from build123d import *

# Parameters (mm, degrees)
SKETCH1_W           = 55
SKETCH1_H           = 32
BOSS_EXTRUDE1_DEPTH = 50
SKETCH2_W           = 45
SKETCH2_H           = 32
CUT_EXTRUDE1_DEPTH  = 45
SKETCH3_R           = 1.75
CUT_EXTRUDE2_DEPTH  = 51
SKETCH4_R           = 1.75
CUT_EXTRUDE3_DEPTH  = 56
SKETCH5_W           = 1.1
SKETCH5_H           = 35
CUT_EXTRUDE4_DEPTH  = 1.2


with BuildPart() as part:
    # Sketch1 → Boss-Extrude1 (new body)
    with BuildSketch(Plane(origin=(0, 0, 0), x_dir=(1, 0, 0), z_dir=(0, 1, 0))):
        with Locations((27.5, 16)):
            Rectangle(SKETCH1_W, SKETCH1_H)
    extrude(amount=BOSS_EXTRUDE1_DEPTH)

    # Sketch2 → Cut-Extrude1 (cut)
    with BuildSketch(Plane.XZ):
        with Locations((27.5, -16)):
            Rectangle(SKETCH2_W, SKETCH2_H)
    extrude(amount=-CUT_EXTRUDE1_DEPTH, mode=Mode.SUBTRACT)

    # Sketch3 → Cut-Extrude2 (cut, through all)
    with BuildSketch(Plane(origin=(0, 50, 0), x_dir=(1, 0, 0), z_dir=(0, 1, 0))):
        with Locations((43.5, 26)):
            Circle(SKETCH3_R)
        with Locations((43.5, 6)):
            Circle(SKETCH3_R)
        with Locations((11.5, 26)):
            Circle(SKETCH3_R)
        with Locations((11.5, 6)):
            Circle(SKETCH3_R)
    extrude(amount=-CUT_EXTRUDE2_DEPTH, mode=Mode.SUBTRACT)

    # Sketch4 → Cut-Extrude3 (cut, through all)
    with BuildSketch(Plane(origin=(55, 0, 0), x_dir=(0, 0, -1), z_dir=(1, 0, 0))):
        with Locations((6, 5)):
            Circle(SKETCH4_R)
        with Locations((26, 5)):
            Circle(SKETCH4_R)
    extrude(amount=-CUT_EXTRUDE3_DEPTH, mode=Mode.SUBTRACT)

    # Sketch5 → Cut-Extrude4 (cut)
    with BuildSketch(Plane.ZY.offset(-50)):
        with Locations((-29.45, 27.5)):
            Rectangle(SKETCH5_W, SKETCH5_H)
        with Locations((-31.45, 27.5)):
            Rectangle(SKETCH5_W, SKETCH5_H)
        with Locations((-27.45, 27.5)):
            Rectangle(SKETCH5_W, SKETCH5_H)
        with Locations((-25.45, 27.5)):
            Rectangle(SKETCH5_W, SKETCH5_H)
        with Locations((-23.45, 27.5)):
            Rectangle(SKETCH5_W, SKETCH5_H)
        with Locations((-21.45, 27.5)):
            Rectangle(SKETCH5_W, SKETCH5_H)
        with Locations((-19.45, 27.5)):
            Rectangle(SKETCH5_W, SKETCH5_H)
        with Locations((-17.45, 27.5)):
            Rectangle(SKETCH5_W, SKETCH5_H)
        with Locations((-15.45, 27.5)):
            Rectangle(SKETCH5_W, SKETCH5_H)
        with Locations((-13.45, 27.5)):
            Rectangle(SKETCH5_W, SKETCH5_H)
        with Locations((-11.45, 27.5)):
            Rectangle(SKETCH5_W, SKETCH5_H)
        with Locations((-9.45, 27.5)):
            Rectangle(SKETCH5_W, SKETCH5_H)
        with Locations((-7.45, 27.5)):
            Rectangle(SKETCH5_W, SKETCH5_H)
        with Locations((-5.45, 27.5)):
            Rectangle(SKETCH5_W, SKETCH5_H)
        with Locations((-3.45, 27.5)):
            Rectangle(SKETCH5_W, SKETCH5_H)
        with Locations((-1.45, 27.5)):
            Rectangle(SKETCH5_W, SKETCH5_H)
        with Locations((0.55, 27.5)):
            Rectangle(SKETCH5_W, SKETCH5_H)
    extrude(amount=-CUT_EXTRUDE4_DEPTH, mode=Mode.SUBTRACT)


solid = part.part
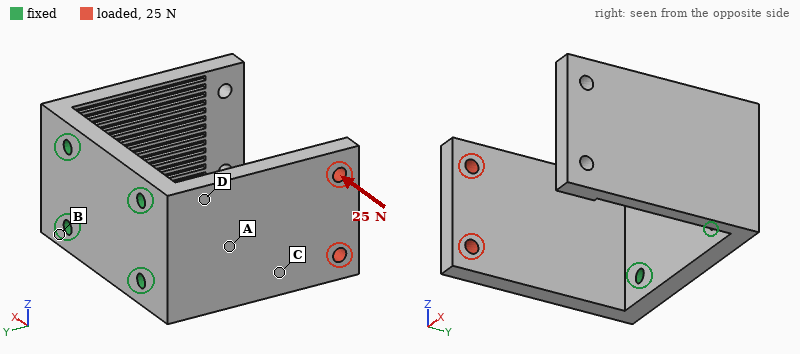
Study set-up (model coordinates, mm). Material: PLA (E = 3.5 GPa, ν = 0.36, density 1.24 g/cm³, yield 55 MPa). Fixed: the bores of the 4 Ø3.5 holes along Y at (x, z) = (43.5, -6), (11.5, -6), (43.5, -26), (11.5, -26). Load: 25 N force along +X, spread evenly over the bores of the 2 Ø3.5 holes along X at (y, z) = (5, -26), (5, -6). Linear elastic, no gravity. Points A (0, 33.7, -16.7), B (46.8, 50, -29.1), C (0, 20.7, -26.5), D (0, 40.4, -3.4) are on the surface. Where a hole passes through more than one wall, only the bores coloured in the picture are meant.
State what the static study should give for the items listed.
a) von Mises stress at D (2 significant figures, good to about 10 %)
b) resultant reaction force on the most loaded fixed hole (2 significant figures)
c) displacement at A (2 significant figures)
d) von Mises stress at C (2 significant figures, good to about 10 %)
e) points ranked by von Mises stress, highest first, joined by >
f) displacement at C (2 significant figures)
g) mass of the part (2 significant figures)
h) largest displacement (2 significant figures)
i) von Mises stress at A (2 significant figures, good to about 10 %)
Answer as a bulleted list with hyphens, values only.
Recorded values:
- 6.5 MPa
- 14 N
- 0.18 mm
- 2.9 MPa
- D > A > C > B
- 0.42 mm
- 27 g
- 0.92 mm
- 4.7 MPa
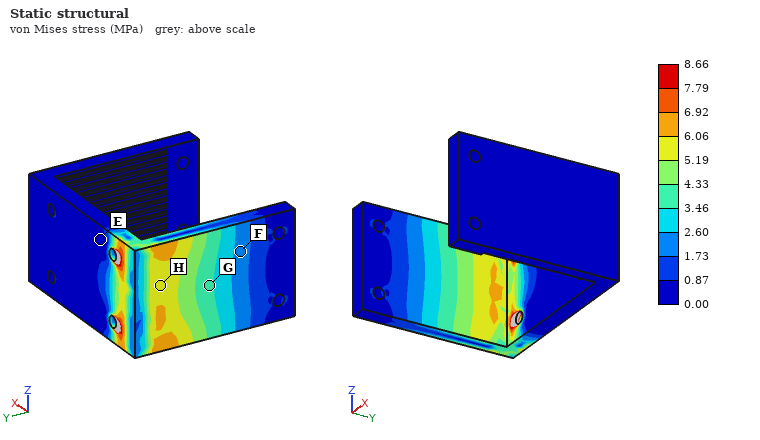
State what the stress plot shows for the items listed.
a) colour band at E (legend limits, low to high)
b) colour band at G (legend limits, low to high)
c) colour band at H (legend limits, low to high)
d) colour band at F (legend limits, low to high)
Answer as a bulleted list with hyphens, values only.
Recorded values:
- 0.00 to 0.87 MPa
- 3.46 to 4.33 MPa
- 5.19 to 6.06 MPa
- 1.73 to 2.60 MPa
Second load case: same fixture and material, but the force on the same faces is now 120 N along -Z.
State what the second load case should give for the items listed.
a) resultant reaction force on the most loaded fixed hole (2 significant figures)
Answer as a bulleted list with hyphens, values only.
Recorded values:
- 240 N
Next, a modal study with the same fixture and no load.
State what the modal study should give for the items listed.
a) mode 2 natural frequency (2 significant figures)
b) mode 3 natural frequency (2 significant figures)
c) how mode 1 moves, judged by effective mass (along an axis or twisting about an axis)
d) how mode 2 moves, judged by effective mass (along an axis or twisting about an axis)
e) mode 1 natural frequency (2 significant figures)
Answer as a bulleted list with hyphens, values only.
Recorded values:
- 490 Hz
- 1200 Hz
- along X
- along X
- 460 Hz
